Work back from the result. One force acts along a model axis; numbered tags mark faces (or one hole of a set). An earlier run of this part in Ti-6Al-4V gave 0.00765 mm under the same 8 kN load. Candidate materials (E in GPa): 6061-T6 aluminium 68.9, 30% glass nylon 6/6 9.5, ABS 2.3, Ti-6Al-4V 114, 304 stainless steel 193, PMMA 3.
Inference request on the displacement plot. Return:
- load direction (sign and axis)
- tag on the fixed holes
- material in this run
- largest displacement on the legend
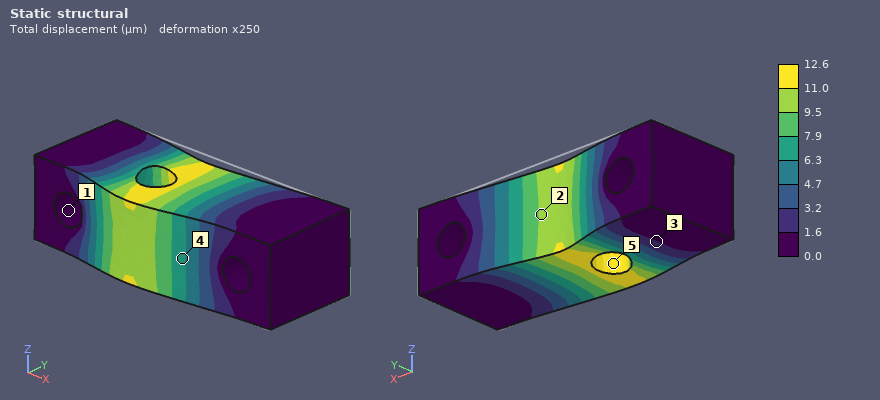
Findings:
-Y
1
6061-T6 aluminium
12.6 µm
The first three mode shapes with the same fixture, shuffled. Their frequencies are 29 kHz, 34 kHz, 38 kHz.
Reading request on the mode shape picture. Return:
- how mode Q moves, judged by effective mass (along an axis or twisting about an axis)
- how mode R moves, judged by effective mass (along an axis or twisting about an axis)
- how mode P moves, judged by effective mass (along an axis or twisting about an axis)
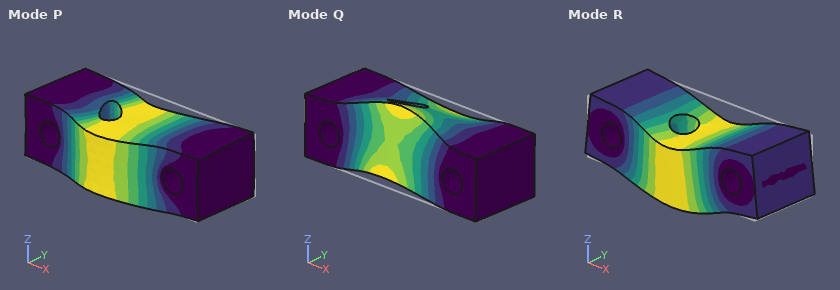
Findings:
twisting about X
along Z
along Y
